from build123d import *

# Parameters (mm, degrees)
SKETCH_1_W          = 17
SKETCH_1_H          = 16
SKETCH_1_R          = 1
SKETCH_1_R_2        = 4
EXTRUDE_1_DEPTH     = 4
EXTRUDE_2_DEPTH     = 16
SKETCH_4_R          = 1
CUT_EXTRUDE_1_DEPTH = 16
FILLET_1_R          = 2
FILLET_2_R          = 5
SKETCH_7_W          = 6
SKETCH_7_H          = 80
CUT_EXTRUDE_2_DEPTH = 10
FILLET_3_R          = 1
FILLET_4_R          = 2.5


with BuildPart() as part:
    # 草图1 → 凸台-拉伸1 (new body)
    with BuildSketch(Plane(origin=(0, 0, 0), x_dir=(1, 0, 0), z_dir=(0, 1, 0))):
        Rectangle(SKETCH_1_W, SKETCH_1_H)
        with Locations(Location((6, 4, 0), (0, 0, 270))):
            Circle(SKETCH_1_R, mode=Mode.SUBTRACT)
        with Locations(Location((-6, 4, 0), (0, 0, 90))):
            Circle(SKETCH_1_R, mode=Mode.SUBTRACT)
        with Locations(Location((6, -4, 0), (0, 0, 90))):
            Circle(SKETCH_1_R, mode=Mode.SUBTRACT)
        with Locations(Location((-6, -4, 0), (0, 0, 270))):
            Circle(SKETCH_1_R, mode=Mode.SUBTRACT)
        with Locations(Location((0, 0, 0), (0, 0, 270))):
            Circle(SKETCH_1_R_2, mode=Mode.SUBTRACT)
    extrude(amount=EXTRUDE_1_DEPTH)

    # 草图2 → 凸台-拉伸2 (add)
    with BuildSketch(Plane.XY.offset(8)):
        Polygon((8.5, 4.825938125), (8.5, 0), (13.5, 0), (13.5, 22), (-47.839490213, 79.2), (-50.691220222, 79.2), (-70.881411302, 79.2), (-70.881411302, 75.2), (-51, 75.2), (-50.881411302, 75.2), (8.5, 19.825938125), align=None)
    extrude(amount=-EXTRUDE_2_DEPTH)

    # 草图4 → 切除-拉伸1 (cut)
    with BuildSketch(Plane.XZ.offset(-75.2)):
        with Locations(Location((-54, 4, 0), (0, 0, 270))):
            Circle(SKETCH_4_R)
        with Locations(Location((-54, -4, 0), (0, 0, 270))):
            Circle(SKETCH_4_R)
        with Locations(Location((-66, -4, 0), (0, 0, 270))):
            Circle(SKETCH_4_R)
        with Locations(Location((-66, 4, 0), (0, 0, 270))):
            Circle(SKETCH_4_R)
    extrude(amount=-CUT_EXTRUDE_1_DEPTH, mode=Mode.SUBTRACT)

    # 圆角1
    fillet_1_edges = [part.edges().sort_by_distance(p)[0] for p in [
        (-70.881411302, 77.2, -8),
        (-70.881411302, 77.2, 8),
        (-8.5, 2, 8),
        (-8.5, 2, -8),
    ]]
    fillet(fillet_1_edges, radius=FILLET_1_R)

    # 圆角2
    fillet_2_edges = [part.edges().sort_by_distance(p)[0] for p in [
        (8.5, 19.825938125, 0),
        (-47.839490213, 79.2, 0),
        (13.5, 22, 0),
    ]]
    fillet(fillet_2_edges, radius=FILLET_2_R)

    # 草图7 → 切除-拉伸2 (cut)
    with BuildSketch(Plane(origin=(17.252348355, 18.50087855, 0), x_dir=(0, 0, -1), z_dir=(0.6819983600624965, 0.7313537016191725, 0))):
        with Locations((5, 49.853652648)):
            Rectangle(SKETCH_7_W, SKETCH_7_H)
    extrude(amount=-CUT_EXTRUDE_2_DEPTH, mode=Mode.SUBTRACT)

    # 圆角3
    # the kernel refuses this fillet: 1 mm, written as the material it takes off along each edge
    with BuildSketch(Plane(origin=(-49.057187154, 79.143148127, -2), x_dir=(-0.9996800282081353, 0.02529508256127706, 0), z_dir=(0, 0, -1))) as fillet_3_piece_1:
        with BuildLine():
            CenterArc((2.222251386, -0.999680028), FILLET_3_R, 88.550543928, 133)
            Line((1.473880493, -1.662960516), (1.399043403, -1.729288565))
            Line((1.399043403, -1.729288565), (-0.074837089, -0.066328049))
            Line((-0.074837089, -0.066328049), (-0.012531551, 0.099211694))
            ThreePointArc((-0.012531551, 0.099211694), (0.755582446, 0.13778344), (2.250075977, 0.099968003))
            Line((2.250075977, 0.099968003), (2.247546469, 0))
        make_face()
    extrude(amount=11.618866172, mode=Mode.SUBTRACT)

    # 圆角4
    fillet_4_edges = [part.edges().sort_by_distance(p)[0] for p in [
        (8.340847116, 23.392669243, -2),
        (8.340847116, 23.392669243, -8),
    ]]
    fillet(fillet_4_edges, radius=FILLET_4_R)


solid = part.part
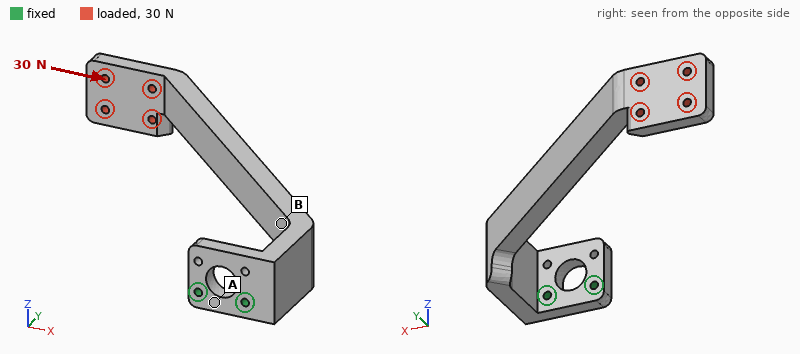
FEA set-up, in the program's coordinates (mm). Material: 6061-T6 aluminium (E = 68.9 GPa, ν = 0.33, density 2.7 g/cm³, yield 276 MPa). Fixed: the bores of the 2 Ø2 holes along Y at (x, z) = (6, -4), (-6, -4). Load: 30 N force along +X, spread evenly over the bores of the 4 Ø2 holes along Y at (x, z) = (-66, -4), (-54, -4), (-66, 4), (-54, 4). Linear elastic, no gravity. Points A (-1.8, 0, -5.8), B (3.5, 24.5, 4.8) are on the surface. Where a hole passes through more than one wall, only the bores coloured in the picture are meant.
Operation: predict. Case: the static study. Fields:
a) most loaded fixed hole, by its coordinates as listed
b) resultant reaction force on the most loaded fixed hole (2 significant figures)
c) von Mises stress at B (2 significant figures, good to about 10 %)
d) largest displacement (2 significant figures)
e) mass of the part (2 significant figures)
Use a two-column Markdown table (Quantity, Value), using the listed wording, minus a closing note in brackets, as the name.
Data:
| Quantity | Value |
|---|---|
| most loaded fixed hole, by its coordinates as listed | (6, -4) |
| resultant reaction force on the most loaded fixed hole | 68 N |
| von Mises stress at B | 35 MPa |
| largest displacement | 1.3 mm |
| mass of the part | 22 g |
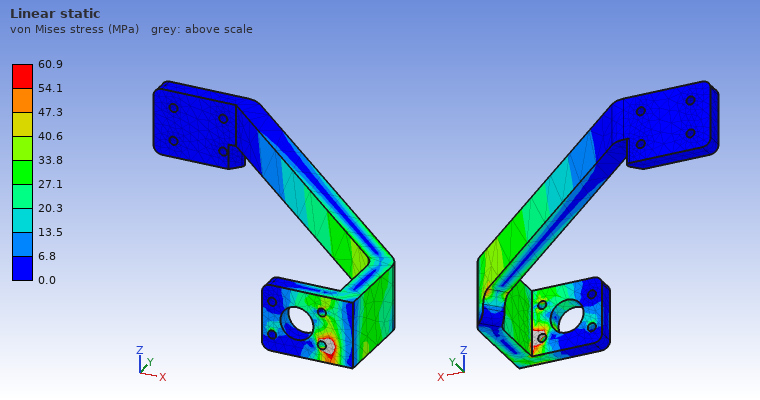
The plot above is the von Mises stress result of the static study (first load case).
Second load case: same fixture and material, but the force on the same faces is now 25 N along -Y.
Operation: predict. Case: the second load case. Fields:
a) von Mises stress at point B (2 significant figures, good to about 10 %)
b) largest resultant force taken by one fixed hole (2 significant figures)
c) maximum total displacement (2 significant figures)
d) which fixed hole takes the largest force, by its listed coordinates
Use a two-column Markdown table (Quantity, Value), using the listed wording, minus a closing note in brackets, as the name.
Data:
| Quantity | Value |
|---|---|
| von Mises stress at point B | 38 MPa |
| largest resultant force taken by one fixed hole | 45 N |
| maximum total displacement | 1.3 mm |
| which fixed hole takes the largest force, by its listed coordinates | (-6, -4) |
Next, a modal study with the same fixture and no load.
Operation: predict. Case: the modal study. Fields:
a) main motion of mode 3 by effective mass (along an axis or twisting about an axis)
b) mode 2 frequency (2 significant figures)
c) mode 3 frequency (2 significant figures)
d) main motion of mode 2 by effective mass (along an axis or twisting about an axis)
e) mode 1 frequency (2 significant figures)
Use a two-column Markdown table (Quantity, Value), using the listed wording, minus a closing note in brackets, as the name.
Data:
| Quantity | Value |
|---|---|
| main motion of mode 3 by effective mass | along X |
| mode 2 frequency | 420 Hz |
| mode 3 frequency | 1500 Hz |
| main motion of mode 2 by effective mass | along Z |
| mode 1 frequency | 270 Hz |
